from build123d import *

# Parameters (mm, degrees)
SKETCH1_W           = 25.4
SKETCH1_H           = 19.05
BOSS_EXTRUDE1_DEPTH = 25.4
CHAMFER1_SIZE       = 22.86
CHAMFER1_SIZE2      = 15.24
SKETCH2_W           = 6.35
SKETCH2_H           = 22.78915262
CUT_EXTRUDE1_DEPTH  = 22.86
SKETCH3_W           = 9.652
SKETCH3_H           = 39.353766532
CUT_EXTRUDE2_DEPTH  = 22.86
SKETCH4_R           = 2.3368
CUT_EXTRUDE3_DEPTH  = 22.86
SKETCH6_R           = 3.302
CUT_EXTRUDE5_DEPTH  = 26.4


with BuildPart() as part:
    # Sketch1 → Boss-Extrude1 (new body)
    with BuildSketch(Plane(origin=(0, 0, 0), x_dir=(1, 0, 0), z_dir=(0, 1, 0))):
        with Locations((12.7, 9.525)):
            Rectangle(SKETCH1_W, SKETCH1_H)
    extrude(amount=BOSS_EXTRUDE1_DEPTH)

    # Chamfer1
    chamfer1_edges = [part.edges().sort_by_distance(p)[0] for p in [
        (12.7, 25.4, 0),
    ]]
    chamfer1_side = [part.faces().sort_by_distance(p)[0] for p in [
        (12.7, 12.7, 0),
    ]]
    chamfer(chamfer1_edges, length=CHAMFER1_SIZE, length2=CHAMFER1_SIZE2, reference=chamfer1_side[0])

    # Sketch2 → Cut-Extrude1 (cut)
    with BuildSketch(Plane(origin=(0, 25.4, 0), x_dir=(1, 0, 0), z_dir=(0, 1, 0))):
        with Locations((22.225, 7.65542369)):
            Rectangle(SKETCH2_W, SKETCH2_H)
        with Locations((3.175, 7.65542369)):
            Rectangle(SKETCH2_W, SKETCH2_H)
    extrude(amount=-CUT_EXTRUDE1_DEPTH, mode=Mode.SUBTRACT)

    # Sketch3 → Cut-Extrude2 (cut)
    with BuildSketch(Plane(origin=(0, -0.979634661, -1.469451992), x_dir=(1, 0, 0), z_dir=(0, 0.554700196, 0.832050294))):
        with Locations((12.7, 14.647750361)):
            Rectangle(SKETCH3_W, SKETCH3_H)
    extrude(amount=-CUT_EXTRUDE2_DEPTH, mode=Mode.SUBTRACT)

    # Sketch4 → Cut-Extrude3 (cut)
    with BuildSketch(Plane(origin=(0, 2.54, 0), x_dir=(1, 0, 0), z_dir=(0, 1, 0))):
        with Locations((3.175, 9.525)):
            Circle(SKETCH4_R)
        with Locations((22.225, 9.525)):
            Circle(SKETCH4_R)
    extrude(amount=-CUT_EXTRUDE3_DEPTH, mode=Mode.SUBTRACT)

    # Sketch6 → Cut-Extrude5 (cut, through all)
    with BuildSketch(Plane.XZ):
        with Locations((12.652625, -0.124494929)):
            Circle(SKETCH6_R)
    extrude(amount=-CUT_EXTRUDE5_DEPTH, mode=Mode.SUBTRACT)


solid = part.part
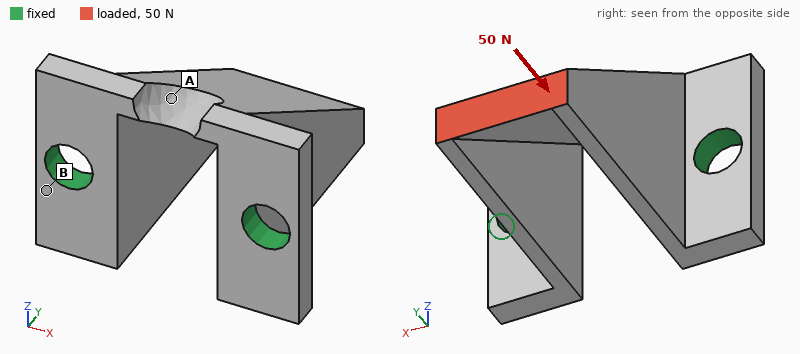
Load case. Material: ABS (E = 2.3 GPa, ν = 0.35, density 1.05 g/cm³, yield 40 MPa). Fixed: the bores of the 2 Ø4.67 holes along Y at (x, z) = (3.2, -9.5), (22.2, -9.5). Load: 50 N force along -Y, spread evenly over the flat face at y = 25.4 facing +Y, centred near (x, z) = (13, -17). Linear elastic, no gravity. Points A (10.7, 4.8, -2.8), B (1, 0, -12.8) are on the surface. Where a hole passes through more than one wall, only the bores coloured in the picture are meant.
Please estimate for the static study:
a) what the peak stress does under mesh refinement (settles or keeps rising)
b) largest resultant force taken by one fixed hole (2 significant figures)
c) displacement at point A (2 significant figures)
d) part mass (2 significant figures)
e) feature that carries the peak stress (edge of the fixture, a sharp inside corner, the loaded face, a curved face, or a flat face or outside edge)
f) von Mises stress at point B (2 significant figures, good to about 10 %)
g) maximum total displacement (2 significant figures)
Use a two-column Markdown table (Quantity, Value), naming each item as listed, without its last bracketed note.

| Quantity | Value |
|---|---|
| what the peak stress does under mesh refinement | keeps rising |
| largest resultant force taken by one fixed hole | 25 N |
| displacement at point A | 0.035 mm |
| part mass | 2.4 g |
| feature that carries the peak stress | edge of the fixture |
| von Mises stress at point B | 3.9 MPa |
| maximum total displacement | 0.23 mm |
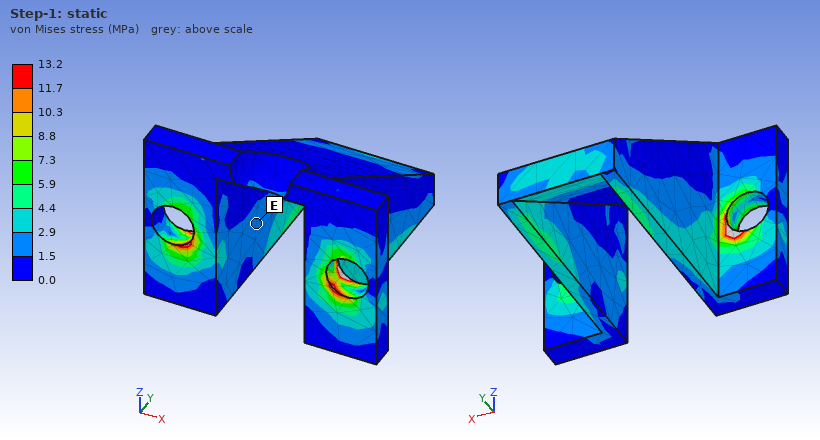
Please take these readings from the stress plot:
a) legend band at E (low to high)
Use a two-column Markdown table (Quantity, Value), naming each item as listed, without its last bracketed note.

| Quantity | Value |
|---|---|
| legend band at E | 1.5 to 2.9 MPa |
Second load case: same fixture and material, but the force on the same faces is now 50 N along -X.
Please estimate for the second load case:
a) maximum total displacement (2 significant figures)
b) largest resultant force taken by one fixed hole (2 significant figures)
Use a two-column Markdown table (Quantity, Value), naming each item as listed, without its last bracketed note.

| Quantity | Value |
|---|---|
| maximum total displacement | 0.48 mm |
| largest resultant force taken by one fixed hole | 89 N |
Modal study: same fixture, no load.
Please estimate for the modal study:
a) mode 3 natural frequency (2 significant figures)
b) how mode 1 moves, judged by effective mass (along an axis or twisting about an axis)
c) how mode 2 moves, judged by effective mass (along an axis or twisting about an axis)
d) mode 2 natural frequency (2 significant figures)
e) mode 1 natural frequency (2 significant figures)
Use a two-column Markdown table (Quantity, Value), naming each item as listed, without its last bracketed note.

| Quantity | Value |
|---|---|
| mode 3 natural frequency | 5600 Hz |
| how mode 1 moves, judged by effective mass | along Z |
| how mode 2 moves, judged by effective mass | along X |
| mode 2 natural frequency | 2300 Hz |
| mode 1 natural frequency | 2100 Hz |
